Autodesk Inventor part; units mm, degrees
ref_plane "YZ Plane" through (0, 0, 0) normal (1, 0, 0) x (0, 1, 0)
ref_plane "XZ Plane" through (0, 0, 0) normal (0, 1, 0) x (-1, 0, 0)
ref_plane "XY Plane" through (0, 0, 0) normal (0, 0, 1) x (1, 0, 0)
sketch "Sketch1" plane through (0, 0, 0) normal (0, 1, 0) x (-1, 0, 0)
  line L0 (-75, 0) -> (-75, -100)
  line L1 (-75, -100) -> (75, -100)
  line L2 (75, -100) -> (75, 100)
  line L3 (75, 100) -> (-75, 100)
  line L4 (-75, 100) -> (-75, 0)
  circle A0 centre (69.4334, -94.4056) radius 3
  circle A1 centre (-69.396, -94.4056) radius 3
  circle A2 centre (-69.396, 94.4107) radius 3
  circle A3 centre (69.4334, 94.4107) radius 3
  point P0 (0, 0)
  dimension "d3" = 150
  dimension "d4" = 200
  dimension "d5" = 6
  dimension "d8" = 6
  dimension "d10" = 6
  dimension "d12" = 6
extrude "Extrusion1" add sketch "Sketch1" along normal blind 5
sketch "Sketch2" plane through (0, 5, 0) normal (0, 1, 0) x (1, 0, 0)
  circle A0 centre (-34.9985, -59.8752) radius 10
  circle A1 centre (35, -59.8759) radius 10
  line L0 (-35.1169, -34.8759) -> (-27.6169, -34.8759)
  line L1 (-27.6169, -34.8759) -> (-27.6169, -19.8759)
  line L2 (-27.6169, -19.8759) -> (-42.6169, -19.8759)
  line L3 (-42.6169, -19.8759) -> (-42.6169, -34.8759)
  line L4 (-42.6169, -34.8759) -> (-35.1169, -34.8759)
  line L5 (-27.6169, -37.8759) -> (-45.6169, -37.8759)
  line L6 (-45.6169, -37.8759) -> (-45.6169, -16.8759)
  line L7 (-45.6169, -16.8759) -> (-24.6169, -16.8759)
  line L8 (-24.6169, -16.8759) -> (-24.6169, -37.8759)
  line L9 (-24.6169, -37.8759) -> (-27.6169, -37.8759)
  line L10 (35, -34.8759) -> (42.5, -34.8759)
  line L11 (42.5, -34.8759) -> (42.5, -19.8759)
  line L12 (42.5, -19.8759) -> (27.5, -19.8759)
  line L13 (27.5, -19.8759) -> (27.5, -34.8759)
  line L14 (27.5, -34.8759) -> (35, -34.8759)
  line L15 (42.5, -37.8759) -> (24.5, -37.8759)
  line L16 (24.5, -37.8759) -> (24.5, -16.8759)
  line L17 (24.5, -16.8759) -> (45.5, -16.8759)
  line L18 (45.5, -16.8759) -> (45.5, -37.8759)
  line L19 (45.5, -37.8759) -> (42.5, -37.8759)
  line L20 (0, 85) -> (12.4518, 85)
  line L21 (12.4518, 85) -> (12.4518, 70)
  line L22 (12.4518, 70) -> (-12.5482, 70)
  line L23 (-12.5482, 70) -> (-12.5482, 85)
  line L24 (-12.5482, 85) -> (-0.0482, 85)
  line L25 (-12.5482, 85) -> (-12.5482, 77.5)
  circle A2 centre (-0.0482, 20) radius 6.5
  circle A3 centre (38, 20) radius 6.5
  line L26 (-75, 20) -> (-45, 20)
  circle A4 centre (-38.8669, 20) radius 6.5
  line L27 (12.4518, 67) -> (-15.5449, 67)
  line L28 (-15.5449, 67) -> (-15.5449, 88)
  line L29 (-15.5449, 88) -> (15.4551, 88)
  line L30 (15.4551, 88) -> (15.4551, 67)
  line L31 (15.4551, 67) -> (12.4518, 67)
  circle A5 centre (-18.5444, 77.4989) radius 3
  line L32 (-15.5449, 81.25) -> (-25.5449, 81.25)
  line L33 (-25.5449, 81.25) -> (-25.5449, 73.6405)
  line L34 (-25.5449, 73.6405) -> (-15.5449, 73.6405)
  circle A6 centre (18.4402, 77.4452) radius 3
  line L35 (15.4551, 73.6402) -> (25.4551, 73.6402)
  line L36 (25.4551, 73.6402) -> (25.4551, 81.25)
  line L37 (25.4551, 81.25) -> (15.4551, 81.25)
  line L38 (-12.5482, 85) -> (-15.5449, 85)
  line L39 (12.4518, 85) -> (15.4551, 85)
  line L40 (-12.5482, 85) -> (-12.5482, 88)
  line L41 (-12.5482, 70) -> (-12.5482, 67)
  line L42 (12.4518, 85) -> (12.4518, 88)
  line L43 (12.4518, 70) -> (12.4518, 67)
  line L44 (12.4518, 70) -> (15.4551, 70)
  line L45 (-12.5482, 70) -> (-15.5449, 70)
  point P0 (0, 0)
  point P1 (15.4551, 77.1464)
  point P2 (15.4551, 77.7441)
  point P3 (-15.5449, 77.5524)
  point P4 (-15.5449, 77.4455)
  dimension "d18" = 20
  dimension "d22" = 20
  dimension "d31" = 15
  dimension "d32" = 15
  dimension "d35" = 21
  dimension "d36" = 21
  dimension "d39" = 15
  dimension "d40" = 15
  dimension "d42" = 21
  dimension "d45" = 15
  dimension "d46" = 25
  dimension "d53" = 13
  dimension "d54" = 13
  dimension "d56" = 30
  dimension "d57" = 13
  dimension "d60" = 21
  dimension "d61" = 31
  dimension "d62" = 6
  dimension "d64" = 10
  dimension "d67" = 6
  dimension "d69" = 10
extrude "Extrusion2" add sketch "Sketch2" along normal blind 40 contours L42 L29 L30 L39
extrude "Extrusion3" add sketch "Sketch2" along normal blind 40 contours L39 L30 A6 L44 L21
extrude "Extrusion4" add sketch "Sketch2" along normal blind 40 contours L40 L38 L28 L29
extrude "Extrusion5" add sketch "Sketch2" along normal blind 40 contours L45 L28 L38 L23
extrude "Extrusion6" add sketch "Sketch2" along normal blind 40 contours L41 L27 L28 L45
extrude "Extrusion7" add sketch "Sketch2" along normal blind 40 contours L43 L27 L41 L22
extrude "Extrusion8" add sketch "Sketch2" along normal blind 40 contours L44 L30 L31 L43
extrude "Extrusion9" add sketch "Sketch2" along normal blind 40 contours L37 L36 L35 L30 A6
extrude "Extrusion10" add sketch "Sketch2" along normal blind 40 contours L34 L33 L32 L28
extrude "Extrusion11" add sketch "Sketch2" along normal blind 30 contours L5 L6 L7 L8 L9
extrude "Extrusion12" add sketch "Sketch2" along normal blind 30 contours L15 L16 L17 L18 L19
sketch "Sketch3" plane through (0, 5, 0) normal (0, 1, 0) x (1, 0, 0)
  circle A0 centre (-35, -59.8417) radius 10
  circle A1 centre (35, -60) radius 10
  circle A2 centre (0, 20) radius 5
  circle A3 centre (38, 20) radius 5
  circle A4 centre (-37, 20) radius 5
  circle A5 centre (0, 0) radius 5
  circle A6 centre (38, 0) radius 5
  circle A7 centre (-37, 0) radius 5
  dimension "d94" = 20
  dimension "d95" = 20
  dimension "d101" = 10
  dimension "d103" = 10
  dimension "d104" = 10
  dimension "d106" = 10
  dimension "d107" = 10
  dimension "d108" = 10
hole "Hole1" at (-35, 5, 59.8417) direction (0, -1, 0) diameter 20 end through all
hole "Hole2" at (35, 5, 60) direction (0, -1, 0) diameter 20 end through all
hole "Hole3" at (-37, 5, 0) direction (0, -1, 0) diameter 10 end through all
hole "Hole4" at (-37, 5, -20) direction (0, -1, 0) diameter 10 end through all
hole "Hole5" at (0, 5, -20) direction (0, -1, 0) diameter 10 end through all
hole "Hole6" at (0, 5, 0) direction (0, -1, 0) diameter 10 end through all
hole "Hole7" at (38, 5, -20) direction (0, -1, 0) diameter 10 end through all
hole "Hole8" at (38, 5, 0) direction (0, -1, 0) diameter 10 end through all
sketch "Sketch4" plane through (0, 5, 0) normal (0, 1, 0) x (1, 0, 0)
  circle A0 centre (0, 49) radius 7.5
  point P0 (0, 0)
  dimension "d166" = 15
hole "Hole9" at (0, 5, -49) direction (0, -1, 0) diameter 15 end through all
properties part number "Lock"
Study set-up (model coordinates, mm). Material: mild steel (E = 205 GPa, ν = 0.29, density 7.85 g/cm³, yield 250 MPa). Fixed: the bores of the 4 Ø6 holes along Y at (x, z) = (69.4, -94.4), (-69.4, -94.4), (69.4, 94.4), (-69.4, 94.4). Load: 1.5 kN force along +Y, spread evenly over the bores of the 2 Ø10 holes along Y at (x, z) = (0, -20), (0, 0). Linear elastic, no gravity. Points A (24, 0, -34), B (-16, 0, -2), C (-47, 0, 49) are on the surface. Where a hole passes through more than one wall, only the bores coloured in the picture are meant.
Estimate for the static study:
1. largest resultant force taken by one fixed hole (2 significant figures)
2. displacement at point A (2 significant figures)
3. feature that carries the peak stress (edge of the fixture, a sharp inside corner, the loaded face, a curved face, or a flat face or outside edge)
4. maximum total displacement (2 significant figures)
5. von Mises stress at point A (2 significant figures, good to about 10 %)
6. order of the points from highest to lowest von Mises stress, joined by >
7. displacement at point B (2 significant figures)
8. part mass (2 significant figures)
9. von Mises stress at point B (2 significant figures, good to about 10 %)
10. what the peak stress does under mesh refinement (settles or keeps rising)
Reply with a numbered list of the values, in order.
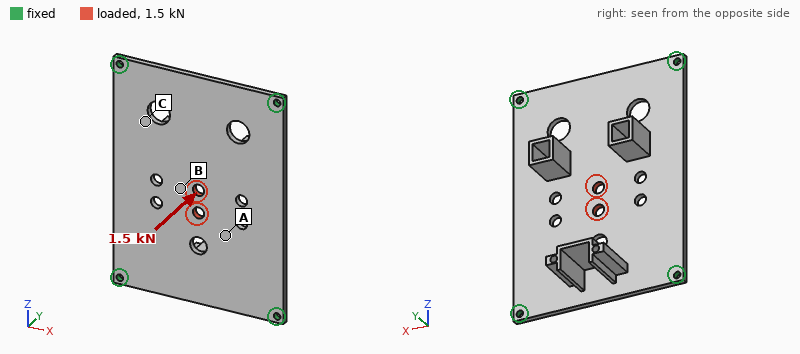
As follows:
1. 430 N
2. 0.27 mm
3. edge of the fixture
4. 0.35 mm
5. 42 MPa
6. B > A > C
7. 0.33 mm
8. 1.3 kg
9. 75 MPa
10. keeps rising
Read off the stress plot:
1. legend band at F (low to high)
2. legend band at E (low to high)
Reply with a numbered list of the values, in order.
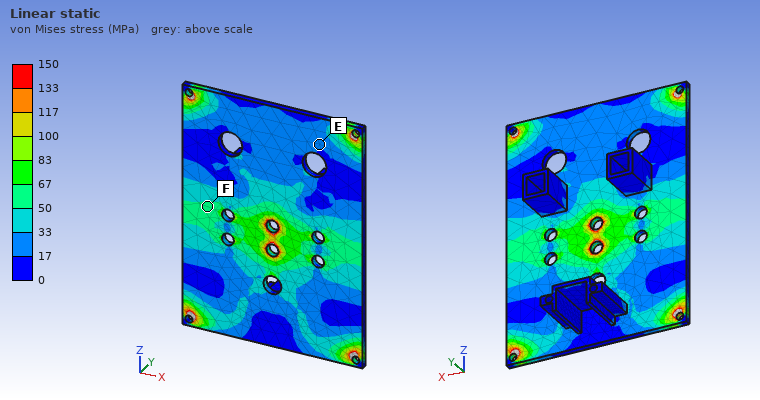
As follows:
1. 50 to 67 MPa
2. 17 to 33 MPa
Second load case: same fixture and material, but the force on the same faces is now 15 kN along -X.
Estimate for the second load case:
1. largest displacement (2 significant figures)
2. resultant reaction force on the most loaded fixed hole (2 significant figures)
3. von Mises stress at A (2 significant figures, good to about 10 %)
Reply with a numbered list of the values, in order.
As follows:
1. 24 µm
2. 5.1 kN
3. 28 MPa
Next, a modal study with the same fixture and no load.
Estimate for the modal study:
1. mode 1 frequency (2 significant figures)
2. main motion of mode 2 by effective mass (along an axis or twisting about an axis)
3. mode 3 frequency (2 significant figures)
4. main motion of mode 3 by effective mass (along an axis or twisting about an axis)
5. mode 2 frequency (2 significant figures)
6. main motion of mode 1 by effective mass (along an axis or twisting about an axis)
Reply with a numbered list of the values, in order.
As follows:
1. 490 Hz
2. twisting about Z
3. 1100 Hz
4. twisting about X
5. 870 Hz
6. along Y
